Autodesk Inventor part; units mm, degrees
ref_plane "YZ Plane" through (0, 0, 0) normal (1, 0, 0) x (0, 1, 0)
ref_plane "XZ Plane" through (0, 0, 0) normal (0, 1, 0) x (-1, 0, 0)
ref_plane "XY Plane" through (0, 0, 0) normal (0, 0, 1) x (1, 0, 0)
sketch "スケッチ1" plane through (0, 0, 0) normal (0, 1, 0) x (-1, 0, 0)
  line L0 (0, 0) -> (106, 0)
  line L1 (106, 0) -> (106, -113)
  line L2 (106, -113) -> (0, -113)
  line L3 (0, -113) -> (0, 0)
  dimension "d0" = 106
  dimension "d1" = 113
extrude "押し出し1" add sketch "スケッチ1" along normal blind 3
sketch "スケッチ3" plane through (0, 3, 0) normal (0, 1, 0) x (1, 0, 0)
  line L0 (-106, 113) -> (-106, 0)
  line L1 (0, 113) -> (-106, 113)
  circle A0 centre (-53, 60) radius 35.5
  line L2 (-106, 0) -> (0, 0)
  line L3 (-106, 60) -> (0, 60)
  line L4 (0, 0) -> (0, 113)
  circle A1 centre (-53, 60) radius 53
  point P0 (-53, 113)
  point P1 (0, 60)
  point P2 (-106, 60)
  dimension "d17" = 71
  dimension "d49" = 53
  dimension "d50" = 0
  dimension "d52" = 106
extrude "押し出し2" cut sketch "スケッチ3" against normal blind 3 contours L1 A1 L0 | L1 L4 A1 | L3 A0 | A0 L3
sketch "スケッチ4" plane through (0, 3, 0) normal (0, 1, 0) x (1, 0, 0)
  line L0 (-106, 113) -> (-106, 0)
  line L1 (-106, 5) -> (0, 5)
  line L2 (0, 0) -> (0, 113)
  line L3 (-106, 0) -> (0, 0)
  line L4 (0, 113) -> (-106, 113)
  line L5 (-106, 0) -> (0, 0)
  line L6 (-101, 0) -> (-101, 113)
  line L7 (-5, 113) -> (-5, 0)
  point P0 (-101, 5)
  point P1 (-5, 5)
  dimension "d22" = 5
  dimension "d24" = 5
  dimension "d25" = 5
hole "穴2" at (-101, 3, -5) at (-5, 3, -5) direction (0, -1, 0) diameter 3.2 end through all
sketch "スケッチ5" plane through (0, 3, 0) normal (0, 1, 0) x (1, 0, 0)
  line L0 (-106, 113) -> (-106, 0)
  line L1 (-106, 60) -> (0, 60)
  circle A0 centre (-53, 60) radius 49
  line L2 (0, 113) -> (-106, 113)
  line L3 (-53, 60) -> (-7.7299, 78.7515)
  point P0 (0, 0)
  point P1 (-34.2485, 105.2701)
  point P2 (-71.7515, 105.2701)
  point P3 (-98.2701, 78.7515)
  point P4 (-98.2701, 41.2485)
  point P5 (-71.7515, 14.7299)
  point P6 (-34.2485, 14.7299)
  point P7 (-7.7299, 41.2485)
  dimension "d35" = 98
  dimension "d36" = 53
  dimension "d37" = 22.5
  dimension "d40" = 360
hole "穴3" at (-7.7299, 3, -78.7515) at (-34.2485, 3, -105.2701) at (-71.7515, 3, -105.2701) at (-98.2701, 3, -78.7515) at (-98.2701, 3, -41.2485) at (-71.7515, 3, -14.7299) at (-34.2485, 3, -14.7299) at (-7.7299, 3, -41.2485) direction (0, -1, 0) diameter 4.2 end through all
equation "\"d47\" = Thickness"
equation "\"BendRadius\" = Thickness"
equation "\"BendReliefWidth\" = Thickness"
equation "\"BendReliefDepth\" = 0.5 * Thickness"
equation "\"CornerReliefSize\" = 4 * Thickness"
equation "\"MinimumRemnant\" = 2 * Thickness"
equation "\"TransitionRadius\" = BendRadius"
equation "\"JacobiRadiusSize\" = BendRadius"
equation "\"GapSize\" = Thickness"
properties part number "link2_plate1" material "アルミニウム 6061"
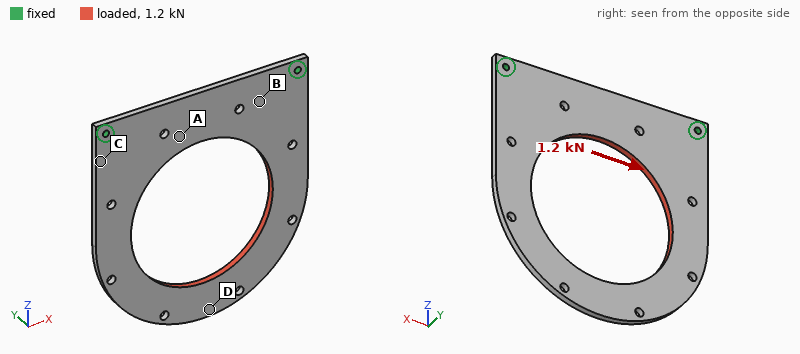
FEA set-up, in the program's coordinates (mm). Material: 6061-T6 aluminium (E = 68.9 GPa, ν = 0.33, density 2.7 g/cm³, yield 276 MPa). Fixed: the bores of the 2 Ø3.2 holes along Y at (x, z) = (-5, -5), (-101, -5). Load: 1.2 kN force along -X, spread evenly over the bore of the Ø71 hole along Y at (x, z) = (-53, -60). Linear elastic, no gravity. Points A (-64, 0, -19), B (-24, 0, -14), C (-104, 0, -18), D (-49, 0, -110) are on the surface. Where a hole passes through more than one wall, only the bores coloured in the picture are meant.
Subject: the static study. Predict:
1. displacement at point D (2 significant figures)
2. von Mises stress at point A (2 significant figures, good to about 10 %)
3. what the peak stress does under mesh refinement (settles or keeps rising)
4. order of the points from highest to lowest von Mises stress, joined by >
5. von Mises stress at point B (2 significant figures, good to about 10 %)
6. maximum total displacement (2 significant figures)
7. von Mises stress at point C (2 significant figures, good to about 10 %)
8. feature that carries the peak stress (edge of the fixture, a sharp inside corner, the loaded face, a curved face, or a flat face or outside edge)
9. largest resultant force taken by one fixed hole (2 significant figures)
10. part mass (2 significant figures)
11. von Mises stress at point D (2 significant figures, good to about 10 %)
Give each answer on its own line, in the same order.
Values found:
0.100 mm
16 MPa
keeps rising
C > A > B > D
8.1 MPa
0.11 mm
21 MPa
edge of the fixture
900 N
54 g
4.4 MPa
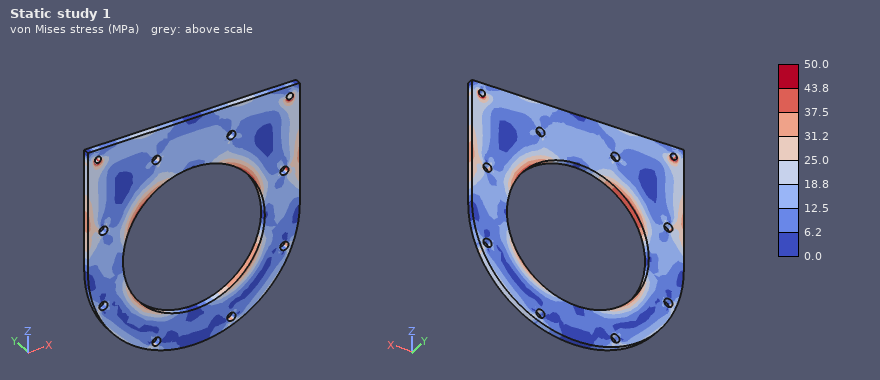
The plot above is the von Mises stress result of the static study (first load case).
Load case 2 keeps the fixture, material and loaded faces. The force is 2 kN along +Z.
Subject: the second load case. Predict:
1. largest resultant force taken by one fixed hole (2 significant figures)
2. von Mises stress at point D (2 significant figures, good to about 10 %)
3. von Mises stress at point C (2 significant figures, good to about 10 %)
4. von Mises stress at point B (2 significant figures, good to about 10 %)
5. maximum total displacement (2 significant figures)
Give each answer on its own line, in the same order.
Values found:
1.0 kN
9.1 MPa
22 MPa
6.6 MPa
30 µm
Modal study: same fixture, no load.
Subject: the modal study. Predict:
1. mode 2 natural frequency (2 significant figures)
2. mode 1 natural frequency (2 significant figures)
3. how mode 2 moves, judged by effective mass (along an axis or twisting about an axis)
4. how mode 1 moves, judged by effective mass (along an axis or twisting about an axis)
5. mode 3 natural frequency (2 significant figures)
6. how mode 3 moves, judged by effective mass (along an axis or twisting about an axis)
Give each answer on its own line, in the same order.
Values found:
570 Hz
200 Hz
twisting about Z
along Y
1100 Hz
along Y
